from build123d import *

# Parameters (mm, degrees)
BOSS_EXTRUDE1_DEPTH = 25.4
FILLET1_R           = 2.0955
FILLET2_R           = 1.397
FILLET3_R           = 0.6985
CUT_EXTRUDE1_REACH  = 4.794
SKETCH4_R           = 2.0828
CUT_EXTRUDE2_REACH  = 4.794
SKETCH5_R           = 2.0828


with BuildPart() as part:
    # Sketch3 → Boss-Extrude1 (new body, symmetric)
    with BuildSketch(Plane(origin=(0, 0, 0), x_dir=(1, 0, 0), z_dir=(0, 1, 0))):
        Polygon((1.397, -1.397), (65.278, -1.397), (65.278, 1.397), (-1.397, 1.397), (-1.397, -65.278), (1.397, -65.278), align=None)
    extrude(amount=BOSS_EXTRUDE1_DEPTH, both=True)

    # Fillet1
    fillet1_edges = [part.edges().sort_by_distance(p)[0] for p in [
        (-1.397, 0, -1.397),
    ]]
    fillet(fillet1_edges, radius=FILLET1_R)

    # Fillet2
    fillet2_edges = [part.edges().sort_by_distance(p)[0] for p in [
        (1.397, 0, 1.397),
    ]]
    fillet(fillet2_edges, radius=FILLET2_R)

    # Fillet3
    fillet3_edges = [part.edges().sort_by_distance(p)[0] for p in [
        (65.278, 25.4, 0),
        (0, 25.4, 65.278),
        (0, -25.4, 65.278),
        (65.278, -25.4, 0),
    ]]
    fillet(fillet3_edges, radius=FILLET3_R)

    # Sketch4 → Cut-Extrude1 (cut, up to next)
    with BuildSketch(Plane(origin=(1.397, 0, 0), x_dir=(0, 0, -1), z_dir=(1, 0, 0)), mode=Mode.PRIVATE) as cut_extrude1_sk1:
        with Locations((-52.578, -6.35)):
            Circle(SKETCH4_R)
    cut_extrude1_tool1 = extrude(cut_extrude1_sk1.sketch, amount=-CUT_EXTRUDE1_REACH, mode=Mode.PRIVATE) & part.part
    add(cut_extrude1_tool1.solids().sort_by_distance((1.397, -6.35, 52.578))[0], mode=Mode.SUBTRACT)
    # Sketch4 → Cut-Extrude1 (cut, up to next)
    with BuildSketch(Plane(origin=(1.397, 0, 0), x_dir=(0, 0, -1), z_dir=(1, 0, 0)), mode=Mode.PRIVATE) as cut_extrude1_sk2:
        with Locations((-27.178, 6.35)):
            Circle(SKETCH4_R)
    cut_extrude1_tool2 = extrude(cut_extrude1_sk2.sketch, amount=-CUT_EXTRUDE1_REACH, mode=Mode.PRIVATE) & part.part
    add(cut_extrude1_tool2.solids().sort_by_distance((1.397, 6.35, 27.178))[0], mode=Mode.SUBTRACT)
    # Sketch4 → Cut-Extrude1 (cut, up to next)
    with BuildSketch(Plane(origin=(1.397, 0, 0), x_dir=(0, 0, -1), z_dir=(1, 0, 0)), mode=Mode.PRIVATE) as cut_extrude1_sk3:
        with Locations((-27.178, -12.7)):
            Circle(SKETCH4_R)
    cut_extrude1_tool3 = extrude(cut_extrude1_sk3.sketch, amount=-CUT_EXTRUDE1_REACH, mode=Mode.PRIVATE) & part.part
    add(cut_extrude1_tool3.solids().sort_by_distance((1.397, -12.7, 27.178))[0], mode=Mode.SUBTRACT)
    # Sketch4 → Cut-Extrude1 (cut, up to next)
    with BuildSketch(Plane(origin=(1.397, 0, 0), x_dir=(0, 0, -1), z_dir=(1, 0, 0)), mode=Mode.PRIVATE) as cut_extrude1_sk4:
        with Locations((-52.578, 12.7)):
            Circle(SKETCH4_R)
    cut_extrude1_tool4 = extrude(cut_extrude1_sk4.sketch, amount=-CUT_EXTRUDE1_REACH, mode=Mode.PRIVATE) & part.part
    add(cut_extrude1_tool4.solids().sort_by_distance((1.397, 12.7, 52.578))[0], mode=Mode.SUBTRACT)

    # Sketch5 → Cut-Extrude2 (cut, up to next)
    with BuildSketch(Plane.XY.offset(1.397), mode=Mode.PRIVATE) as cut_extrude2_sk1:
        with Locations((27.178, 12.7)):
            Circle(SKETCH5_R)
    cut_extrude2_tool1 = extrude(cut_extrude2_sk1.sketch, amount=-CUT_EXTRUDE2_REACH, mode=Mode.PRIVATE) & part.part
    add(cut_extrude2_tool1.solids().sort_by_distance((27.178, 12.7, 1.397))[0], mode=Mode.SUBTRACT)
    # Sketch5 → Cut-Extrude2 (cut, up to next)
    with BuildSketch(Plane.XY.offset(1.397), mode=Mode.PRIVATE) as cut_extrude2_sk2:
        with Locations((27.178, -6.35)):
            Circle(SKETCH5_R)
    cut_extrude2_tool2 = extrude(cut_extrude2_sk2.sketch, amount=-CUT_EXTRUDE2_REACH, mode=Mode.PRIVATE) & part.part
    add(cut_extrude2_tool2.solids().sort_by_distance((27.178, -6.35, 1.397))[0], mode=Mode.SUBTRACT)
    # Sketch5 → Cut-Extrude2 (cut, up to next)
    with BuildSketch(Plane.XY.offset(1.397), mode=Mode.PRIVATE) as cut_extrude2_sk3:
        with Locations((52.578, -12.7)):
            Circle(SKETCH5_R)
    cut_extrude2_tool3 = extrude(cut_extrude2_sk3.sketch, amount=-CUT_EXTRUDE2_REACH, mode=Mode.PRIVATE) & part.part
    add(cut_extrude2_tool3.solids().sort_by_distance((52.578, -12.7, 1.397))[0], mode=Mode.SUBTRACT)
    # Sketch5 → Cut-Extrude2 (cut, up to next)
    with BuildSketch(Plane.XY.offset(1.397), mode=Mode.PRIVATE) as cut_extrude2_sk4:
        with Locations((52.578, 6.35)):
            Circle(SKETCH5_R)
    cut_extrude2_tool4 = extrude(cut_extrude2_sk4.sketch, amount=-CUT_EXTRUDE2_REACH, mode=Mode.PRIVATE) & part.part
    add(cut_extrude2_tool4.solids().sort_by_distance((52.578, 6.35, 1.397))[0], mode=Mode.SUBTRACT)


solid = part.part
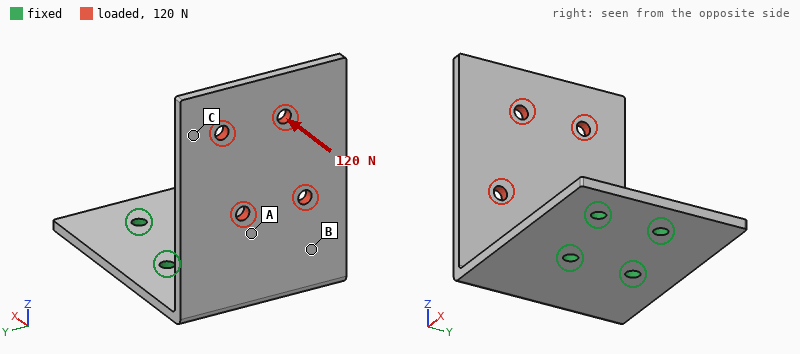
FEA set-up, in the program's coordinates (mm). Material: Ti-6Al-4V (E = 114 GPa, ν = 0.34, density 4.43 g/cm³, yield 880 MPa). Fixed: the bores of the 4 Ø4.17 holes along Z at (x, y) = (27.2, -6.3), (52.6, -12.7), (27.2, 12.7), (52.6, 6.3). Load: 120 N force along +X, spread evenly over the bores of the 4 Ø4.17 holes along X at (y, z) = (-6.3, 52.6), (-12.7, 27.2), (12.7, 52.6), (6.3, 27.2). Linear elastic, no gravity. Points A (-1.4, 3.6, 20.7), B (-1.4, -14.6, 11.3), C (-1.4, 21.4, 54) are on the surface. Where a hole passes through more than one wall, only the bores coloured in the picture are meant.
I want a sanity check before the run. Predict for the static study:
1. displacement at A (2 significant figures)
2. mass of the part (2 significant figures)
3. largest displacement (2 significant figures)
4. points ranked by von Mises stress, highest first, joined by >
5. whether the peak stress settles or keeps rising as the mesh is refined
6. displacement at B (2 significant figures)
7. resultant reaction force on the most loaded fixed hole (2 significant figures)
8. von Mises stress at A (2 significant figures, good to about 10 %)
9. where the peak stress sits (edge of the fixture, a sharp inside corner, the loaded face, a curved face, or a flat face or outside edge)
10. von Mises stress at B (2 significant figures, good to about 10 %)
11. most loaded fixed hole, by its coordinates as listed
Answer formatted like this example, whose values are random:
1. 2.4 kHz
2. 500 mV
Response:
1. 0.35 mm
2. 81 g
3. 1.2 mm
4. B > A > C
5. keeps rising
6. 0.23 mm
7. 76 N
8. 30 MPa
9. edge of the fixture
10. 46 MPa
11. (27.2, -6.3)
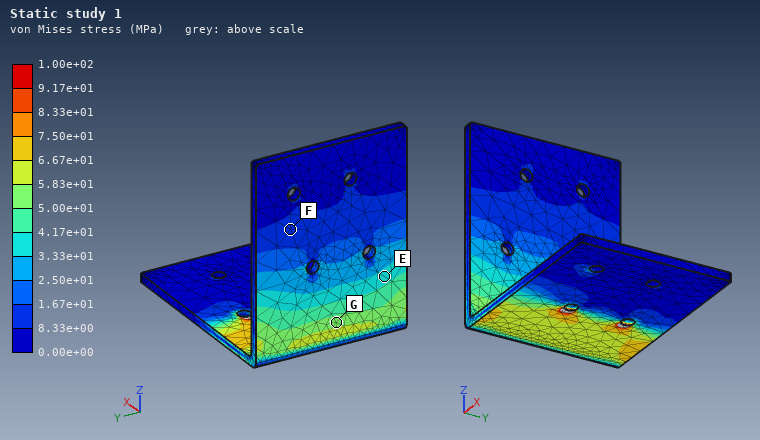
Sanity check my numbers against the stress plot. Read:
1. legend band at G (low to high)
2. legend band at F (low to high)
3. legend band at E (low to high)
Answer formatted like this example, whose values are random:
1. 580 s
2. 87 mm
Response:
1. 5.00e+01 to 5.83e+01 MPa
2. 8.33e+00 to 1.67e+01 MPa
3. 3.33e+01 to 4.17e+01 MPa
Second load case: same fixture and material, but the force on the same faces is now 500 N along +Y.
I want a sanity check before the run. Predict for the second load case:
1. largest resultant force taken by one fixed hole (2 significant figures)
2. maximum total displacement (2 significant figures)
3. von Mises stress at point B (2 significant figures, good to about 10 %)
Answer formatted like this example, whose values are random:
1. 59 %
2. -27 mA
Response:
1. 920 N
2. 1.3 mm
3. 56 MPa
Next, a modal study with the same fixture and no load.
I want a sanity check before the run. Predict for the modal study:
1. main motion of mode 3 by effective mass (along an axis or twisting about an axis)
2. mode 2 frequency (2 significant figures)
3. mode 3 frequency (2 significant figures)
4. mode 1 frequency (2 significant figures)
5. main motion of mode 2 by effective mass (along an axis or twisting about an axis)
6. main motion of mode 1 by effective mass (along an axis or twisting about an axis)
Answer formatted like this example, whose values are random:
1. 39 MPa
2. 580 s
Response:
1. along Z
2. 640 Hz
3. 1300 Hz
4. 340 Hz
5. along Y
6. along X
